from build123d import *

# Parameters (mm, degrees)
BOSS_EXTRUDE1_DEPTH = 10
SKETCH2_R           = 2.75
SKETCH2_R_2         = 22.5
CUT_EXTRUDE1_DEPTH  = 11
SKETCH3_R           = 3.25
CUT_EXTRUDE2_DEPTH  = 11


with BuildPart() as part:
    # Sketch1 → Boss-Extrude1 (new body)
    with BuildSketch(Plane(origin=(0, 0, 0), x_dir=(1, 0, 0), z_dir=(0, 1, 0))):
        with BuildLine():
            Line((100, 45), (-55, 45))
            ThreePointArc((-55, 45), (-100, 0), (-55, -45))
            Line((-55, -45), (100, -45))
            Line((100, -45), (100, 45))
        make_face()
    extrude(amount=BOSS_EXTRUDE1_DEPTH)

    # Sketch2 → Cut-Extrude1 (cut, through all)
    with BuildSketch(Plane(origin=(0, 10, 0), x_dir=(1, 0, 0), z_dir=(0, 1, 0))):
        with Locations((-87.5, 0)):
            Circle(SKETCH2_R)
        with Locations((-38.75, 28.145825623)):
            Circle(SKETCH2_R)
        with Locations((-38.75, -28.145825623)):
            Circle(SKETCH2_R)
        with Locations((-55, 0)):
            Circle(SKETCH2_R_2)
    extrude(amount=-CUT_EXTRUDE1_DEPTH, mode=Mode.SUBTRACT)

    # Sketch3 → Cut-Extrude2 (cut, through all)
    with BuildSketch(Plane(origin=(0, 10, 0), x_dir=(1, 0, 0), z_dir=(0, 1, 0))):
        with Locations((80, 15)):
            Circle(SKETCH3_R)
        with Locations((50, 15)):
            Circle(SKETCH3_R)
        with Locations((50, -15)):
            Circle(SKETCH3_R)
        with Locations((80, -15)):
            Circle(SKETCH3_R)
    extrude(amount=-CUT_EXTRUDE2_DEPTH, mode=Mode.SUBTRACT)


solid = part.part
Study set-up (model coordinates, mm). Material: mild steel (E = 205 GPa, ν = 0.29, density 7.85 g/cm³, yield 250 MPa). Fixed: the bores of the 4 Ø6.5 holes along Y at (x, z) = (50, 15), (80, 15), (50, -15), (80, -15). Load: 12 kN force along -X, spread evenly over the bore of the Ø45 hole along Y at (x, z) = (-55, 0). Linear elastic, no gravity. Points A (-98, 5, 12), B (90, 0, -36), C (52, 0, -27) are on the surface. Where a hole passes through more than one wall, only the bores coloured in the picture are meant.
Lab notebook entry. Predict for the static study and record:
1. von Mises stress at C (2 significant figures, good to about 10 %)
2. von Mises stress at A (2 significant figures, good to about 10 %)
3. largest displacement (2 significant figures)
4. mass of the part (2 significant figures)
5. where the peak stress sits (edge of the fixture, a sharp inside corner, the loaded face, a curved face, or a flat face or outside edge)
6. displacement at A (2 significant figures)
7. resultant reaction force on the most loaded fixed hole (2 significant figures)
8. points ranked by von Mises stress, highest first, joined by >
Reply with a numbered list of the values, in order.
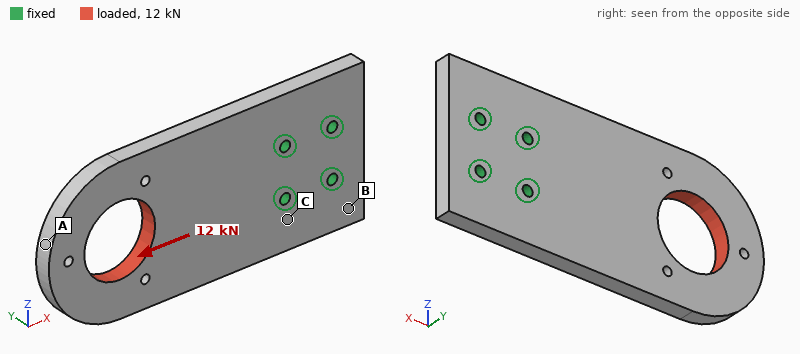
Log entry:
1. 10 MPa
2. 18 MPa
3. 15 µm
4. 1.2 kg
5. a curved face
6. 13 µm
7. 4.7 kN
8. A > C > B
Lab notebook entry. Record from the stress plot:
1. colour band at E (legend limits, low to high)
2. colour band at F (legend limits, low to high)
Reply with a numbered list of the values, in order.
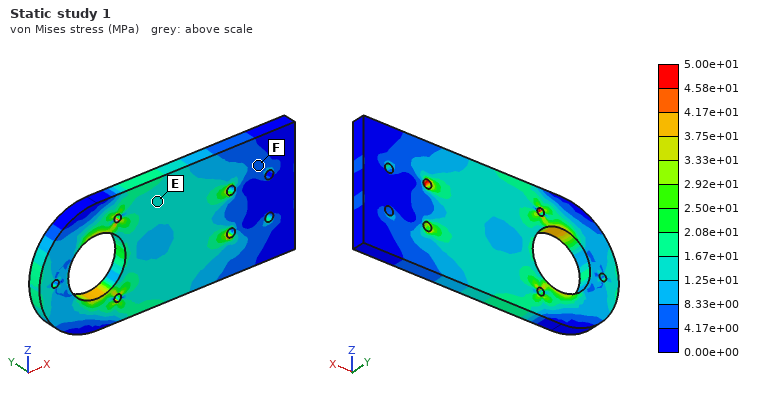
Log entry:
1. 1.25e+01 to 1.67e+01 MPa
2. 4.17e+00 to 8.33e+00 MPa
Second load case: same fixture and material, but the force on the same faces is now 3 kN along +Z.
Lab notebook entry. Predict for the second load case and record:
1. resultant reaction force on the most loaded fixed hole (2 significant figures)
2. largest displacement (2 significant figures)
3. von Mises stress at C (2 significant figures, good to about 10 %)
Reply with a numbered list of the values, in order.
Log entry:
1. 5.3 kN
2. 37 µm
3. 16 MPa
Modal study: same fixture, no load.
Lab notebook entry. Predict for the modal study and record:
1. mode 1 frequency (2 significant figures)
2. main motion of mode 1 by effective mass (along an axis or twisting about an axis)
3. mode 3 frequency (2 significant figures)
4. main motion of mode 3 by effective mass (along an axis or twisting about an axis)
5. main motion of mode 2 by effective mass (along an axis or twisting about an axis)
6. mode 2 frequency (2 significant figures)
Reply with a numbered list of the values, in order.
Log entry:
1. 450 Hz
2. along Y
3. 2100 Hz
4. along Y
5. twisting about X
6. 1400 Hz
